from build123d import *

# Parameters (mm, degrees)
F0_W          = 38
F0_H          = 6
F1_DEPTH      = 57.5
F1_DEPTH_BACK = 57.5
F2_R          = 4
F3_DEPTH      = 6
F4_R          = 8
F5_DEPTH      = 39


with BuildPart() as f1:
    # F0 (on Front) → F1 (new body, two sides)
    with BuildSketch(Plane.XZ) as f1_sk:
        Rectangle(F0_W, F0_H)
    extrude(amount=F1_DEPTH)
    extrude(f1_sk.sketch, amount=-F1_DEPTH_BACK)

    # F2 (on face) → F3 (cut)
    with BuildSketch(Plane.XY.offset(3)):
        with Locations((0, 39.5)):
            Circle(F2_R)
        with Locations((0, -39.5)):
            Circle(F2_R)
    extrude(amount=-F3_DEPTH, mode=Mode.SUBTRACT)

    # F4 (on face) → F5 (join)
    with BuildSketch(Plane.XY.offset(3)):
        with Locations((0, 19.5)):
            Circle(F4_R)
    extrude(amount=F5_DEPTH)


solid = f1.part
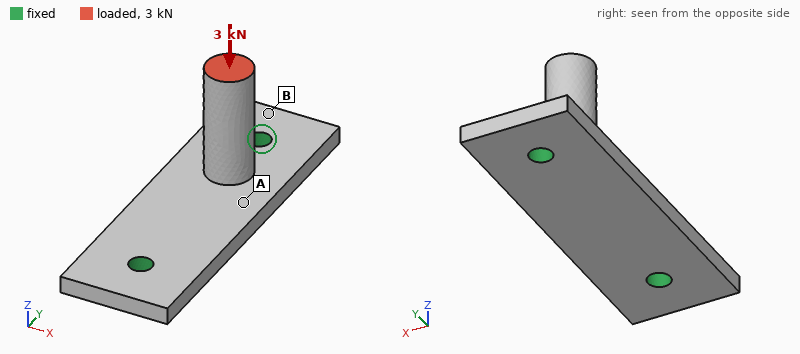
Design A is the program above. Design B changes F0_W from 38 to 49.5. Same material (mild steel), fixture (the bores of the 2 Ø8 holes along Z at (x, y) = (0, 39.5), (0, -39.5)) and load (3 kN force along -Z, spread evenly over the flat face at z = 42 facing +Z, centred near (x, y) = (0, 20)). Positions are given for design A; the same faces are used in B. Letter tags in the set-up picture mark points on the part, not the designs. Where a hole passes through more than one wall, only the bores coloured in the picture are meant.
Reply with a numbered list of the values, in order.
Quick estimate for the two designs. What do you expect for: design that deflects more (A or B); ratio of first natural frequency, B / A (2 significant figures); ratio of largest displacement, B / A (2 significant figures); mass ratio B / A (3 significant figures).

1. A
2. 1.0
3. 0.89
4. 1.24
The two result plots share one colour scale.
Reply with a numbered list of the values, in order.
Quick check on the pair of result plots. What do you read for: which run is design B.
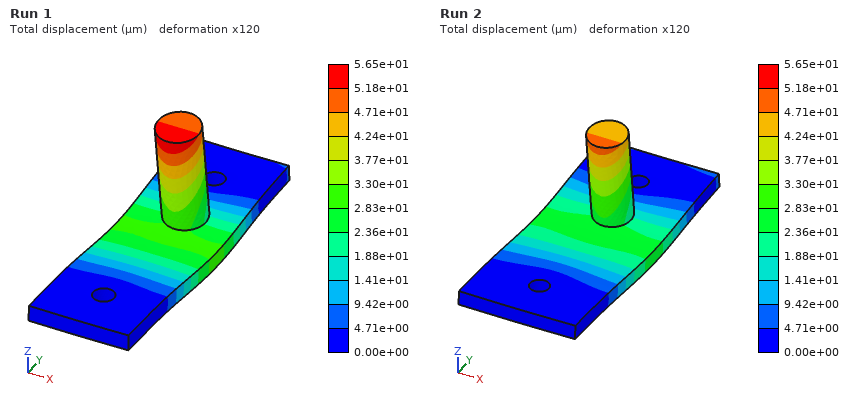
1. Run 2
